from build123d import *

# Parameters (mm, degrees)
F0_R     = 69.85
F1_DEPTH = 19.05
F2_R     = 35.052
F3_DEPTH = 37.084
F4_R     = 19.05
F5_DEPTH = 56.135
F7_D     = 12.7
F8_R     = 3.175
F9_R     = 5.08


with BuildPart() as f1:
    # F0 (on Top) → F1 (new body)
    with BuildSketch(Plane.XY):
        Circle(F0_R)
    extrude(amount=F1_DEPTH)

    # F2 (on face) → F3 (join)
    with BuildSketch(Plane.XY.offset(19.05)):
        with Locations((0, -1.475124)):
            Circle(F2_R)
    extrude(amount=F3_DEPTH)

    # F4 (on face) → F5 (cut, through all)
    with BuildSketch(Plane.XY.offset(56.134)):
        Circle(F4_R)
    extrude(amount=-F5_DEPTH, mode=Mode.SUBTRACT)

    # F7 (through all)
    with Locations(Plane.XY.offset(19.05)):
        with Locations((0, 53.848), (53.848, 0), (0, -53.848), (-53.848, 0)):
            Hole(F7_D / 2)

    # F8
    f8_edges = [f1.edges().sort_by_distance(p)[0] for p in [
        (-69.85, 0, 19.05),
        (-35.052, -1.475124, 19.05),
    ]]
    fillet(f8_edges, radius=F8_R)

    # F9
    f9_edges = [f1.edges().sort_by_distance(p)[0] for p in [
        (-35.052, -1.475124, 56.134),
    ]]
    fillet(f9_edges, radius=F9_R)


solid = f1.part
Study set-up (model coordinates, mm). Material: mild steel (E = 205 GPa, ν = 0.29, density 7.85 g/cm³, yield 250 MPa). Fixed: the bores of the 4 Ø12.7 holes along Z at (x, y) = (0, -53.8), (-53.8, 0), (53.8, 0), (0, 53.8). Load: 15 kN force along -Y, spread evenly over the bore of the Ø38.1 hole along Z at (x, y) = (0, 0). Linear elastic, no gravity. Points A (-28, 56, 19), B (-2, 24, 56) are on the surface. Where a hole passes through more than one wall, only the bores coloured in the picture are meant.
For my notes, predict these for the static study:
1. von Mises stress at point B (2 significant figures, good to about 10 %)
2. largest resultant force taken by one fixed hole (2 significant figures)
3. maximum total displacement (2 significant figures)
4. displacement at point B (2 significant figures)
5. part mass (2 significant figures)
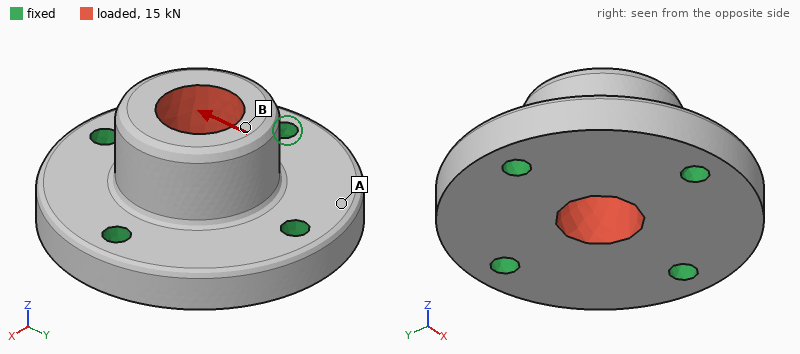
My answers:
5.8 MPa
5.6 kN
4.8 µm
4.7 µm
2.8 kg
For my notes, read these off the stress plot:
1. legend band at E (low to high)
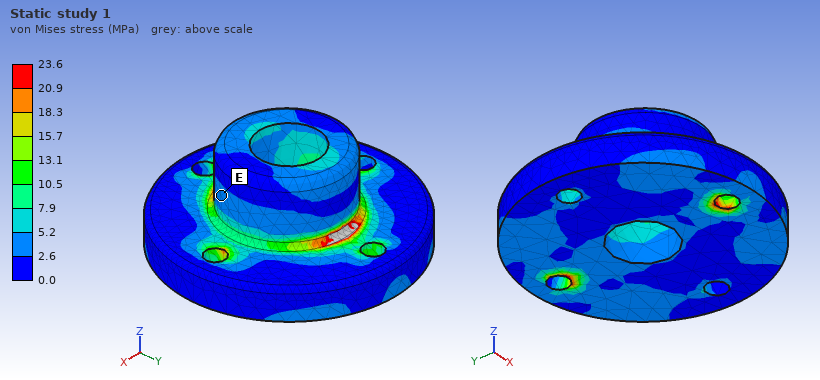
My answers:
2.6 to 5.2 MPa
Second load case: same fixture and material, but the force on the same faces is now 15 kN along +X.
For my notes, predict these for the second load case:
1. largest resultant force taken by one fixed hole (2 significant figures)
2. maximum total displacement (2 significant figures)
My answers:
5.4 kN
4.6 µm
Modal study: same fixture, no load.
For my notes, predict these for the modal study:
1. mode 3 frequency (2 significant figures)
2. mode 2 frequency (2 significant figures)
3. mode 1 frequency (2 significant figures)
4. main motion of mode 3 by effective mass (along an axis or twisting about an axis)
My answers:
9700 Hz
9000 Hz
9000 Hz
along Z
